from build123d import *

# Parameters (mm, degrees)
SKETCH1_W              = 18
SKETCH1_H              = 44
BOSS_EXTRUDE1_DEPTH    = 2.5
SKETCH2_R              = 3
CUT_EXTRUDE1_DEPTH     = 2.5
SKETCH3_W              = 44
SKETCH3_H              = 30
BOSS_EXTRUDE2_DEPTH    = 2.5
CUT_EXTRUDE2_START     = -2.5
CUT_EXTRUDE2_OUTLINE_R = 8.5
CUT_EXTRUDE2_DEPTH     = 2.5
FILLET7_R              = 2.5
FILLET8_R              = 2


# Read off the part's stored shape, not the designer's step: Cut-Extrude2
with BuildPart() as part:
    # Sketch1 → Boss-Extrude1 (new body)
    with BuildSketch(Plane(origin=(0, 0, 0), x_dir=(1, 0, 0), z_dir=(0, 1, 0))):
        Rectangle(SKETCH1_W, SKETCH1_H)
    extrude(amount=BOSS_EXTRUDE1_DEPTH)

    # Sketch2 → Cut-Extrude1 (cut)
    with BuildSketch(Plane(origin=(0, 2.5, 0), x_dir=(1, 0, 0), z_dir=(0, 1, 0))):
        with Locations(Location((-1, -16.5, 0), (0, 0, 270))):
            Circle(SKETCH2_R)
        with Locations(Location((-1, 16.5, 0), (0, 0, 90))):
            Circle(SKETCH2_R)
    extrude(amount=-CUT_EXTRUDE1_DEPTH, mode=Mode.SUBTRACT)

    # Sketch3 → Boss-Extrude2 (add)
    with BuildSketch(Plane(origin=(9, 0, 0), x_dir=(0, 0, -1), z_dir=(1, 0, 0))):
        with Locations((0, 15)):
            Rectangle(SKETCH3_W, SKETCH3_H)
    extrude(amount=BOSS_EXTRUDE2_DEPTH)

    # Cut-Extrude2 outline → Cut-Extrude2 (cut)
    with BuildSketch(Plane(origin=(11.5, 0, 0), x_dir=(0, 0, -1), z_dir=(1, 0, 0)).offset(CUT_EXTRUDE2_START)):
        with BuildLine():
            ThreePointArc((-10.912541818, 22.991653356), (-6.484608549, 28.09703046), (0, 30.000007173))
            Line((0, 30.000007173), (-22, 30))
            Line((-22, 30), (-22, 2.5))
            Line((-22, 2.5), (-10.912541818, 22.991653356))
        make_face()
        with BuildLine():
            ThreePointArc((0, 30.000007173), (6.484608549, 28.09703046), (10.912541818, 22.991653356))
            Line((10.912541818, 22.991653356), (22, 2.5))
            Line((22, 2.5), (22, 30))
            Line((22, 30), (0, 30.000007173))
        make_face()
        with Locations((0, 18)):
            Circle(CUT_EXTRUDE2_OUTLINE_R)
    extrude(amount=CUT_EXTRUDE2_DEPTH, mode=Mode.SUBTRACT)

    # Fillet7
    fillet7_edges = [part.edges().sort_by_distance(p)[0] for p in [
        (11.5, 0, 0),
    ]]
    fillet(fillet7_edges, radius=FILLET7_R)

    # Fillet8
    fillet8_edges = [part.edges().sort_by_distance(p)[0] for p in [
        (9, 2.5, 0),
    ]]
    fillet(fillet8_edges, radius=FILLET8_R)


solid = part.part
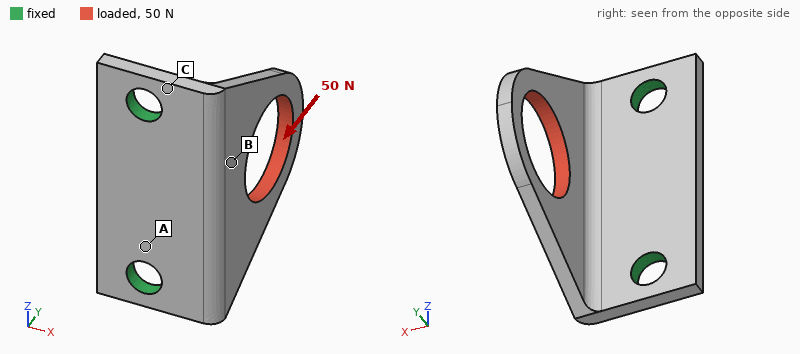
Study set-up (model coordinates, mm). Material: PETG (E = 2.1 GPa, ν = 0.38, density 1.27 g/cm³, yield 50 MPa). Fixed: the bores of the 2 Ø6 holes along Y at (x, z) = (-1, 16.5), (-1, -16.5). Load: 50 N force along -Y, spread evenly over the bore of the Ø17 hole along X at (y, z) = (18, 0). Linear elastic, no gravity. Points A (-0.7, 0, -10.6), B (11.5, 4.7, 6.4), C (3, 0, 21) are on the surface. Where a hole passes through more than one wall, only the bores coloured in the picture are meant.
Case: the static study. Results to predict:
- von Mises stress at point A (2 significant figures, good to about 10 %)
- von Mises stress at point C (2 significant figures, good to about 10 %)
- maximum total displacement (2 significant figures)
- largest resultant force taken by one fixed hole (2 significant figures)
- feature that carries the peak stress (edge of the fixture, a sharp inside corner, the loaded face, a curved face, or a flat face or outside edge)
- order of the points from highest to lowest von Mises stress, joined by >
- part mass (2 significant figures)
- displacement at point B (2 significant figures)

3.6 MPa
8.2 MPa
0.59 mm
25 N
a flat face or outside edge
C > A > B
4.4 g
0.19 mm
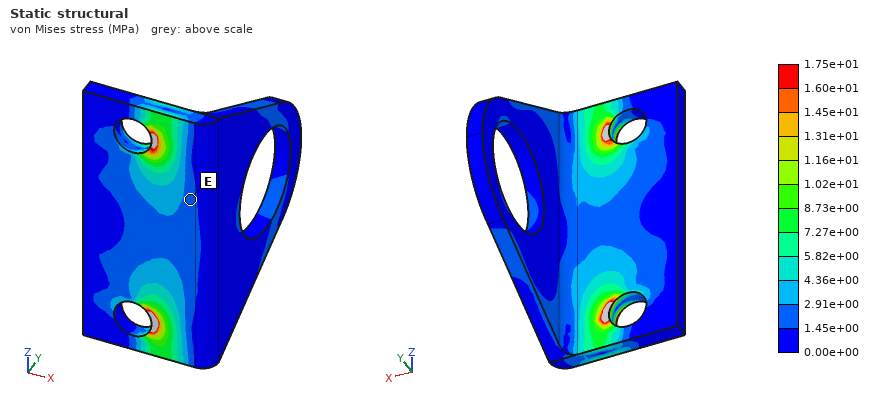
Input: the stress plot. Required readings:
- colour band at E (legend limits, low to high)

1.45e+00 to 2.91e+00 MPa
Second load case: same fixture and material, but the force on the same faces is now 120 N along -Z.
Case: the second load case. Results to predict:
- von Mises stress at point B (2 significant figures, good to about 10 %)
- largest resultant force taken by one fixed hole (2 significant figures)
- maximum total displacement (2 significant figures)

4.0 MPa
91 N
0.65 mm
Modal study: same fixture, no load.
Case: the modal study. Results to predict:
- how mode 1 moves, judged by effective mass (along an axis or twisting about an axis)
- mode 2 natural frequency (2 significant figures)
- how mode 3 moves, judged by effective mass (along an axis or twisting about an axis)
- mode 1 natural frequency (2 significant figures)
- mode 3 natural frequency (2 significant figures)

along X
1700 Hz
along Y
750 Hz
2100 Hz
